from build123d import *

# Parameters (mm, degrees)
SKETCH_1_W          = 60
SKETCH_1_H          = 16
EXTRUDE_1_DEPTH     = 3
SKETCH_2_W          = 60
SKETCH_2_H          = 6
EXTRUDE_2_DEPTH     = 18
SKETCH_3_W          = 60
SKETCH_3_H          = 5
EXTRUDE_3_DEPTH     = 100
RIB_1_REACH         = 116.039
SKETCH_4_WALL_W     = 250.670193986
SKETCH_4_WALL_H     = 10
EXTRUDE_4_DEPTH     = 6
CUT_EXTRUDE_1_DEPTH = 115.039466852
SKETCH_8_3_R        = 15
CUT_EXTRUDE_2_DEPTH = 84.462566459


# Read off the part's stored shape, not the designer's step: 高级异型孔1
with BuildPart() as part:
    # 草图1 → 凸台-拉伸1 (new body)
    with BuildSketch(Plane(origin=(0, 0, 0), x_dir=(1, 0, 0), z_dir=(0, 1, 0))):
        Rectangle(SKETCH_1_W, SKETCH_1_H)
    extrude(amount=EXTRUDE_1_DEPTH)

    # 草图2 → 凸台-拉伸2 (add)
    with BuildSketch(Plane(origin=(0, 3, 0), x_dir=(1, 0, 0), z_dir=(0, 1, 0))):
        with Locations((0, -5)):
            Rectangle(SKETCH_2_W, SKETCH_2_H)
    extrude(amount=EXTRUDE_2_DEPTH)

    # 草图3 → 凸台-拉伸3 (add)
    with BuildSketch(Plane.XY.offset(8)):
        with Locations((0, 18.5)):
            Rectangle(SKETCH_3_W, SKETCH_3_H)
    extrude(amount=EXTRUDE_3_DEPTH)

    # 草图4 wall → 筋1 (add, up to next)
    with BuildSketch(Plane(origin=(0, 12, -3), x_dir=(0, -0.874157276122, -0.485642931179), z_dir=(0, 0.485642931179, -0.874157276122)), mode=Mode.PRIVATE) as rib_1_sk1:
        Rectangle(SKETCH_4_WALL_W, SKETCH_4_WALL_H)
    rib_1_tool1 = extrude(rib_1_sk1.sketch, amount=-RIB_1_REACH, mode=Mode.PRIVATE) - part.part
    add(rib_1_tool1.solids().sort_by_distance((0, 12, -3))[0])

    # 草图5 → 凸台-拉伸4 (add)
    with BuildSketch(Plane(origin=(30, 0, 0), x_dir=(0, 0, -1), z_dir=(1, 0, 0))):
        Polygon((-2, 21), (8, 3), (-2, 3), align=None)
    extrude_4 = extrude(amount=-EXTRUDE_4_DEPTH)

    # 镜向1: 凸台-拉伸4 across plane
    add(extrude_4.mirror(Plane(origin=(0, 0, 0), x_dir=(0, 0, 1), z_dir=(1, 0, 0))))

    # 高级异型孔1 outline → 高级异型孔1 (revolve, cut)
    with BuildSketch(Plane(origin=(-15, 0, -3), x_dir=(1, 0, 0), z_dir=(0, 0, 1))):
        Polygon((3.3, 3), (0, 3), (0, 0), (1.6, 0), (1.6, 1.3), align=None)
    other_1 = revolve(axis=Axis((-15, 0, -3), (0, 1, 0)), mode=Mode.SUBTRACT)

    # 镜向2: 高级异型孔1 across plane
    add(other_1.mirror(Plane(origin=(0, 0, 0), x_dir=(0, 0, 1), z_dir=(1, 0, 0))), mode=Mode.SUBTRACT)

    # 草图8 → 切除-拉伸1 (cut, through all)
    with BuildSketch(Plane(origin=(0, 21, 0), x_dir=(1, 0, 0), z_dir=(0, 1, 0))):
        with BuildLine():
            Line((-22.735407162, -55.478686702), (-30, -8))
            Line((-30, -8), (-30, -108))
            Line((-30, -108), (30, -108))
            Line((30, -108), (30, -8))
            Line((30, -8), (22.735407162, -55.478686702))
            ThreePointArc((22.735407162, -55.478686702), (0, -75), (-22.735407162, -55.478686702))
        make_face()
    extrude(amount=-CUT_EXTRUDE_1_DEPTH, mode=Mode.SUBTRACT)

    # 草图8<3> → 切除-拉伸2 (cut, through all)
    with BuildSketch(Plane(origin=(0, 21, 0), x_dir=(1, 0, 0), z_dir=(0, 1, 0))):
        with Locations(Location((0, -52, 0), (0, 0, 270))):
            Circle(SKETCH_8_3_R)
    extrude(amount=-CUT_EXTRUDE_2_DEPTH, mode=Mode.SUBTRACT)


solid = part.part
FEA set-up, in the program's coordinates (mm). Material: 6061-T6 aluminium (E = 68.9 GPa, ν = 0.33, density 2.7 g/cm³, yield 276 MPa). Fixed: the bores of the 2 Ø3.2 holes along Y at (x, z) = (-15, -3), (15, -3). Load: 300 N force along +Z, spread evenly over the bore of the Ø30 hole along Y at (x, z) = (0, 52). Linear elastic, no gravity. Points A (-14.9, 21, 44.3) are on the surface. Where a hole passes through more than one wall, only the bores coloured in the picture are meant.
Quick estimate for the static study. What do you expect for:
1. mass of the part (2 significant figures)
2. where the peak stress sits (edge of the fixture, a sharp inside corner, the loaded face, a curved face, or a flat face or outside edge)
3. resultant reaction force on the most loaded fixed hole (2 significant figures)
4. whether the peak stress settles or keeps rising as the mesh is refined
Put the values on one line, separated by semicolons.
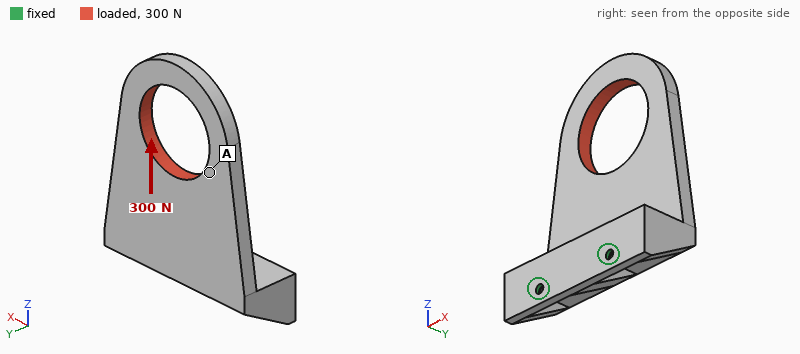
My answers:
64 g; edge of the fixture; 150 N; keeps rising
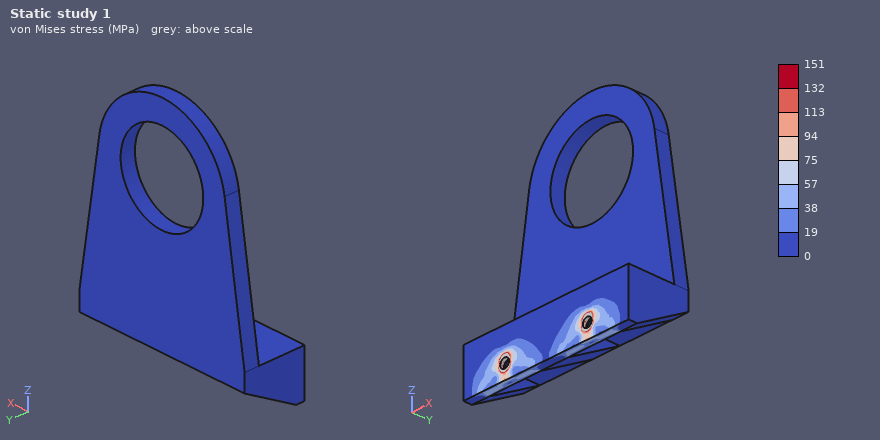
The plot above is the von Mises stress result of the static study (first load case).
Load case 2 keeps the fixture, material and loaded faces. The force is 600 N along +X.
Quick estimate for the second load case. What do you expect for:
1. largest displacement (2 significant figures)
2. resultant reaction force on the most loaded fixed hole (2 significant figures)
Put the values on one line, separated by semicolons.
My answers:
0.19 mm; 1.1 kN
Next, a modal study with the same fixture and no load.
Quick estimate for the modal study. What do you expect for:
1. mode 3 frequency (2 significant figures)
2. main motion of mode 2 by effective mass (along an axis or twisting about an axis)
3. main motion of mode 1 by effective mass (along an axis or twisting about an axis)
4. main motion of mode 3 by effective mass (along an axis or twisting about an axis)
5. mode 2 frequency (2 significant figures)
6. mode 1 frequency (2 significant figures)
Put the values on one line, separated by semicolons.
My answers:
2300 Hz; along X; along Y; along Z; 2200 Hz; 490 Hz
